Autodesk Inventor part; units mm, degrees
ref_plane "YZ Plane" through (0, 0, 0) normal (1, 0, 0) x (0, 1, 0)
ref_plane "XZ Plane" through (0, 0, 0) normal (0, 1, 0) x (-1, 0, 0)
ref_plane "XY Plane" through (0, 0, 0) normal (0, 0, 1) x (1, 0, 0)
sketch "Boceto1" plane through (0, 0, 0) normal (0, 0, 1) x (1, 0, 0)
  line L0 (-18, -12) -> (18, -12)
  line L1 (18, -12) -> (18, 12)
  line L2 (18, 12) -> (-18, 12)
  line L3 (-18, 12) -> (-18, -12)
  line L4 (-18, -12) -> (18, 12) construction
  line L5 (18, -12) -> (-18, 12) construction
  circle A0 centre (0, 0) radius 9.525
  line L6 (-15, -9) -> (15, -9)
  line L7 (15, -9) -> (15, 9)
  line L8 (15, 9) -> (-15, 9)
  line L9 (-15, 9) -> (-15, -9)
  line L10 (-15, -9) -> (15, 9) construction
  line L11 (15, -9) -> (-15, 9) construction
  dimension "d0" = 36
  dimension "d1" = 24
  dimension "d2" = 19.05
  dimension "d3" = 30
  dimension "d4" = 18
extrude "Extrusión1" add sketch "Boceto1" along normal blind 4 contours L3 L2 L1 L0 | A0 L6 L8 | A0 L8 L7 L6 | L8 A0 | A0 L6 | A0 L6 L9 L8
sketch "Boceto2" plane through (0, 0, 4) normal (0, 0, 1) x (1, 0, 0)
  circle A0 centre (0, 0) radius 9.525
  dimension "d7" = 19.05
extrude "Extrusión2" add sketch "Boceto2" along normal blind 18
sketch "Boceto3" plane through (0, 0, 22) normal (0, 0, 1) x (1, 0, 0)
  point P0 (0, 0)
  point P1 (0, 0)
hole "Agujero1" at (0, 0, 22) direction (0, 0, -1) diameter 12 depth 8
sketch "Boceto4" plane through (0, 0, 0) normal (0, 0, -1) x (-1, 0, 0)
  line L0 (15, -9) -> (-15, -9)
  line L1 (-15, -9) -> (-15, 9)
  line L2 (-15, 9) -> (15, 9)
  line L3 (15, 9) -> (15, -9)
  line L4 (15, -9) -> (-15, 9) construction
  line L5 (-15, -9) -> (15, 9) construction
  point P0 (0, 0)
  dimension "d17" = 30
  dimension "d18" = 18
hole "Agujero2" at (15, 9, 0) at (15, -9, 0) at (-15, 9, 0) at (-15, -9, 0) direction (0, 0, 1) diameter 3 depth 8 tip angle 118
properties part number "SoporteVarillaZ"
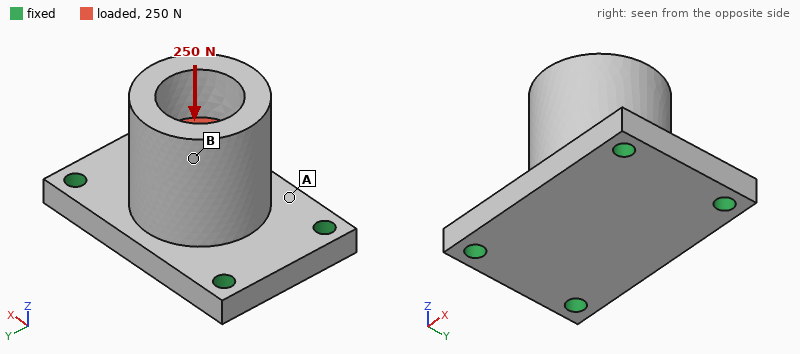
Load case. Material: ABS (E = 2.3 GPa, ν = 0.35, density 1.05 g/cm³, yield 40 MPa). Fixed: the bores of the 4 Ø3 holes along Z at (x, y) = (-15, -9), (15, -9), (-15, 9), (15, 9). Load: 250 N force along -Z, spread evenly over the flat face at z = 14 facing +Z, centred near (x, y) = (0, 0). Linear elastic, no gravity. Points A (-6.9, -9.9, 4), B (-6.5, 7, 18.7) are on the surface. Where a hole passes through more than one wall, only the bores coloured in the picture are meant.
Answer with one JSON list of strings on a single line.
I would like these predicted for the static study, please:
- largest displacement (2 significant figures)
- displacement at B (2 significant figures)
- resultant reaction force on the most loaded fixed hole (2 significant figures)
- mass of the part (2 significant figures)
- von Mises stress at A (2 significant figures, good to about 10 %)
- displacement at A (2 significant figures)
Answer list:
["61 µm", "56 µm", "66 N", "7.9 g", "3.1 MPa", "41 µm"]
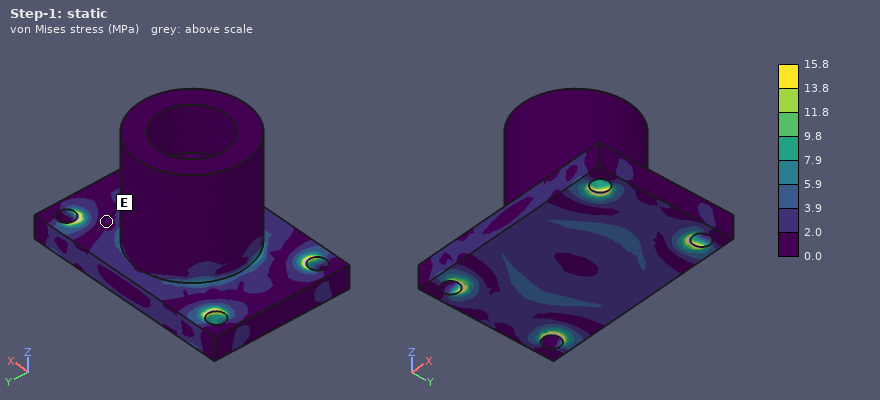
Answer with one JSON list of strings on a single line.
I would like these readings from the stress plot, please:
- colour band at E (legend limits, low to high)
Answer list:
["0.0 to 2.0 MPa"]
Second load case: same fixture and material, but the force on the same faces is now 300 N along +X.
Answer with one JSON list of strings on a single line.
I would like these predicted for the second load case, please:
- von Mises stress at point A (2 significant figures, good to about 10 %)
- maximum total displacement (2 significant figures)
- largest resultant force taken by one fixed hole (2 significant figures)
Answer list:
["5.9 MPa", "0.14 mm", "110 N"]
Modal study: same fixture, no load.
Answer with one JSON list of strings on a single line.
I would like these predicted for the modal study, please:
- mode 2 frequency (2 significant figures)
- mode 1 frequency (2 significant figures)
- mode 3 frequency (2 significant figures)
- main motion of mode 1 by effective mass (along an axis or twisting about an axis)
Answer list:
["4200 Hz", "2900 Hz", "4300 Hz", "along Y"]
